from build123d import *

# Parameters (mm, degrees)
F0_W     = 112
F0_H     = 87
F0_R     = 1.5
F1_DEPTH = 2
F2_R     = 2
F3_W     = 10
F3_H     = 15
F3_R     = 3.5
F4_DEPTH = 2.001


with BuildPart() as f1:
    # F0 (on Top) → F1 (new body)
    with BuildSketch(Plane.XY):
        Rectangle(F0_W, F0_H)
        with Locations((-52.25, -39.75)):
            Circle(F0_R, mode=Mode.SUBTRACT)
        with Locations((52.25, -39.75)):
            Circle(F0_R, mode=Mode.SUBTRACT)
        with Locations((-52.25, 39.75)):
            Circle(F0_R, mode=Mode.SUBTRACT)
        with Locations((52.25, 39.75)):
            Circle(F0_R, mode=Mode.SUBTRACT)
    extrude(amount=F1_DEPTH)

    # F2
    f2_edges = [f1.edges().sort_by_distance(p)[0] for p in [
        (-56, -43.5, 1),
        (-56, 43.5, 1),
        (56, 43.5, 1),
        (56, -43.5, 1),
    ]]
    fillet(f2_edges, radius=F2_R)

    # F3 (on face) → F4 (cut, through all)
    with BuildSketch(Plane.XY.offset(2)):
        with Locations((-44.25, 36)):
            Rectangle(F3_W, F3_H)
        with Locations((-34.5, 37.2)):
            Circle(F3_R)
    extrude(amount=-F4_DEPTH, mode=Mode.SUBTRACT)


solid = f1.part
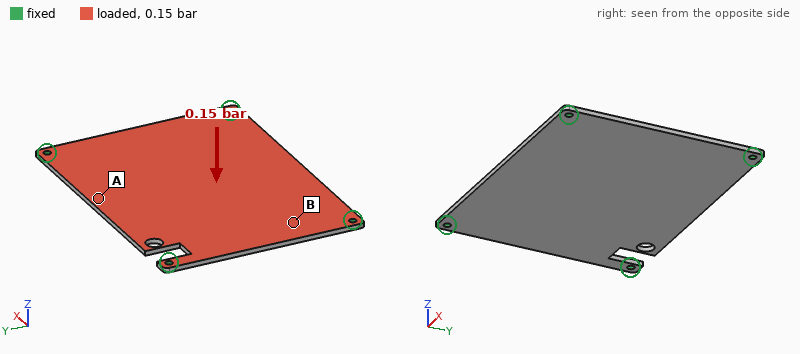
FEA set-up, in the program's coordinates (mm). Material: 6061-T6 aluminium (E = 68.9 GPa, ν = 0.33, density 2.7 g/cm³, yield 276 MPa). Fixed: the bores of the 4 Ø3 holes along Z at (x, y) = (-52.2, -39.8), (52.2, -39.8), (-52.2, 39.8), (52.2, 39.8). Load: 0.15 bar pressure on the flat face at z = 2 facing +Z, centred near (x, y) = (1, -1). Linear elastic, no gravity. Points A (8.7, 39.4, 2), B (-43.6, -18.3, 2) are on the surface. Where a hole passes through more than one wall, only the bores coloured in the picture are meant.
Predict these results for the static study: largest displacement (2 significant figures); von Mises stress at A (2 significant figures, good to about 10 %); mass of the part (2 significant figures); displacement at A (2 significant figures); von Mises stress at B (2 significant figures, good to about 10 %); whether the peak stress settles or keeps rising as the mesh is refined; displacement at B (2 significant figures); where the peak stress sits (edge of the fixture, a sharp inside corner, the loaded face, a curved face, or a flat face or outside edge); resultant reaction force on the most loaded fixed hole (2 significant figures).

0.25 mm
16 MPa
51 g
0.22 mm
5.2 MPa
keeps rising
0.080 mm
edge of the fixture
40 N
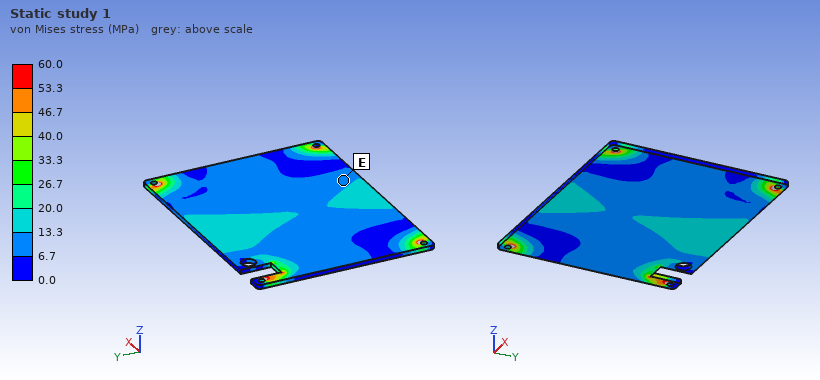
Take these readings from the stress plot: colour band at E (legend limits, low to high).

6.7 to 13.3 MPa
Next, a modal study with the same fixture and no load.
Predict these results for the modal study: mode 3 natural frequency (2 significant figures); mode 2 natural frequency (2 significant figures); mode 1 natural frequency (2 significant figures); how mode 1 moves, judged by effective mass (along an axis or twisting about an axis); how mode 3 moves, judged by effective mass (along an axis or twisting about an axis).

1500 Hz
1000 Hz
620 Hz
along Z
twisting about Y
